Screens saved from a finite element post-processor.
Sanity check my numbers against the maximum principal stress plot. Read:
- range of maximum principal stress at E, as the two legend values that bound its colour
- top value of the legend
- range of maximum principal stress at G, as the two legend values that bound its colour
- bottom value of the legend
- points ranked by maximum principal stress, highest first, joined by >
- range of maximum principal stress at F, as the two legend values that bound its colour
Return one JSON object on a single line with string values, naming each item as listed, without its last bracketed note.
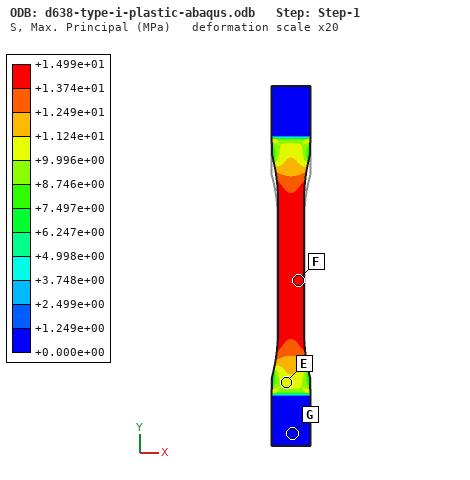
{"range of maximum principal stress at E, as the two legend values that bound its colour": "+9.996e+00 to +1.124e+01 MPa", "top value of the legend": "+1.499e+01 MPa", "range of maximum principal stress at G, as the two legend values that bound its colour": "+0.000e+00 to +1.249e+00 MPa", "bottom value of the legend": "+0.000e+00 MPa", "points ranked by maximum principal stress, highest first, joined by >": "F > E > G", "range of maximum principal stress at F, as the two legend values that bound its colour": "+1.374e+01 to +1.499e+01 MPa"}
